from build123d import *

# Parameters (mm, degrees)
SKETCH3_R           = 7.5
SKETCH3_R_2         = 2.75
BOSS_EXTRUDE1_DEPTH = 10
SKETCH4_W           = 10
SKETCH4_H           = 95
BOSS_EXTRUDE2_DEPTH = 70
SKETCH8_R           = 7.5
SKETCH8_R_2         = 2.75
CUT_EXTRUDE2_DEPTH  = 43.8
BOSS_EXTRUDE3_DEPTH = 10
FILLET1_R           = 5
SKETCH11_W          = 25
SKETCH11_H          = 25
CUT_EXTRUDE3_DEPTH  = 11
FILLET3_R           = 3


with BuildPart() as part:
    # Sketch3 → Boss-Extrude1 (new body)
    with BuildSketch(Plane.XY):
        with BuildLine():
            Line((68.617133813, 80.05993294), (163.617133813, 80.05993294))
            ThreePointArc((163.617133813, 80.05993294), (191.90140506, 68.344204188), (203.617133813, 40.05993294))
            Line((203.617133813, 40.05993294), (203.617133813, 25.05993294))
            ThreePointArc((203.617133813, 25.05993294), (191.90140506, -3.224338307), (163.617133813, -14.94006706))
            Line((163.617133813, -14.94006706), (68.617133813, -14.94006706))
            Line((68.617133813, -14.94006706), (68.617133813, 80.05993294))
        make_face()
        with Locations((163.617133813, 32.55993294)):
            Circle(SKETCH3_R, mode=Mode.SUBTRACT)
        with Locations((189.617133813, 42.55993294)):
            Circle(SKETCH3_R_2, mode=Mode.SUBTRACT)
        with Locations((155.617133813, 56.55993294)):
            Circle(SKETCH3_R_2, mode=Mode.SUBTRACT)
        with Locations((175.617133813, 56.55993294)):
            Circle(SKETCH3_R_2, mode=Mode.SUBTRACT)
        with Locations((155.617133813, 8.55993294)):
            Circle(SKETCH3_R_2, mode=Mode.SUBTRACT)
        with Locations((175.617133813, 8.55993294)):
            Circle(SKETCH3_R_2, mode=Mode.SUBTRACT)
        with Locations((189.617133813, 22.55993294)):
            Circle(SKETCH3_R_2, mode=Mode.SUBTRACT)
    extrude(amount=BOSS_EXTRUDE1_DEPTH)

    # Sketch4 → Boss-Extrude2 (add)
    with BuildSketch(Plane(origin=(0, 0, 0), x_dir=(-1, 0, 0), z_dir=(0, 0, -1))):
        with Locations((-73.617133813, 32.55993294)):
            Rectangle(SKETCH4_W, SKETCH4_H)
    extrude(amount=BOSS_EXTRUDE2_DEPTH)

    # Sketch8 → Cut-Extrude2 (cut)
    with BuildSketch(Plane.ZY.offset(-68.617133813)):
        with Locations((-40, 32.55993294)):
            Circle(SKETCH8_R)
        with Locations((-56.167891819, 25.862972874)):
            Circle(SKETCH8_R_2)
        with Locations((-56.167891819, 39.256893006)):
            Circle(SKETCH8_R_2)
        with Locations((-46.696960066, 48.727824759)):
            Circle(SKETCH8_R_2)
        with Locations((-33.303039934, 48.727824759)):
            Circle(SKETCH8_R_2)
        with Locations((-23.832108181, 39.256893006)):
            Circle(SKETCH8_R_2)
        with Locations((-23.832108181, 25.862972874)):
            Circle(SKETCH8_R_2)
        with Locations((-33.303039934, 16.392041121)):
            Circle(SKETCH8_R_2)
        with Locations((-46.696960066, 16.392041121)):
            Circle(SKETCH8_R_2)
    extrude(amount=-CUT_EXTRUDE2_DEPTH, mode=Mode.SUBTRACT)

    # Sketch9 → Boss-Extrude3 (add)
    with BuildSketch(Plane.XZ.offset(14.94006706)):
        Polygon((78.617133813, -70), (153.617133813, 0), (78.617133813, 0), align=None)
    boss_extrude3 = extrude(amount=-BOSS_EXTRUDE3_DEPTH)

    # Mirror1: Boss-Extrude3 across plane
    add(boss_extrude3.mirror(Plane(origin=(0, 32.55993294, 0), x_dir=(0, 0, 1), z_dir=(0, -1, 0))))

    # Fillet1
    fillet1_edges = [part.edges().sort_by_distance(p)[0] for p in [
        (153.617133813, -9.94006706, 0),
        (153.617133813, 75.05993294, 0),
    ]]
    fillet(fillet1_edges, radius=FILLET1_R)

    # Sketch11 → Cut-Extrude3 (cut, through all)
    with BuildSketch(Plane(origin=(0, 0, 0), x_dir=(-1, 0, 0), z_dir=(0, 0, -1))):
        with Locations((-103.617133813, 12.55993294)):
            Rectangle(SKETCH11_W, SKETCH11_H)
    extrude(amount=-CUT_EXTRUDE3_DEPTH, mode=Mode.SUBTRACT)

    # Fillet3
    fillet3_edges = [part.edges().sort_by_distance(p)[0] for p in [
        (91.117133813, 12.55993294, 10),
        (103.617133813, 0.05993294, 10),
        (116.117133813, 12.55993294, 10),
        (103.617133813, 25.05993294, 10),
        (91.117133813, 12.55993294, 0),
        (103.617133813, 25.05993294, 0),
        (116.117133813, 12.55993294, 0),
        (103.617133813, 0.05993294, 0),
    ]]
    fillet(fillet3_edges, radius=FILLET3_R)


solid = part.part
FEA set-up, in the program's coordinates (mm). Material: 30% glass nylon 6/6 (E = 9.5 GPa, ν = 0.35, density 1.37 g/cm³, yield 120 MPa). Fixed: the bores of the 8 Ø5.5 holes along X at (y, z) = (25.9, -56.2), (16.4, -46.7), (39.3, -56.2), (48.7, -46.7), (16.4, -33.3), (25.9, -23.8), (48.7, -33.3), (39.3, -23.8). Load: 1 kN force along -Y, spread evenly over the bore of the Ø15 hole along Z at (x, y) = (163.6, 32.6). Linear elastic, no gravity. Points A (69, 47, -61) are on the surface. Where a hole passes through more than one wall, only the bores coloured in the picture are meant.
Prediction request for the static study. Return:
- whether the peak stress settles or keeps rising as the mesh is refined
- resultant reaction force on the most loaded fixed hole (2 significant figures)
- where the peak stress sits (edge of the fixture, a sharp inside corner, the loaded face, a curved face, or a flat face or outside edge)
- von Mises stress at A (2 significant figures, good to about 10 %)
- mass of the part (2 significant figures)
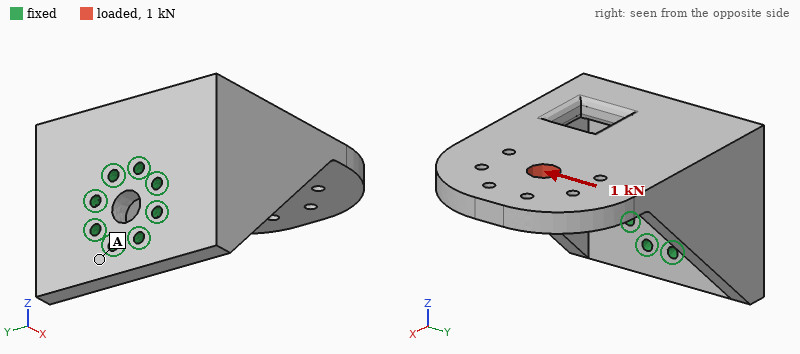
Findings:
keeps rising
1.1 kN
edge of the fixture
6.4 MPa
310 g
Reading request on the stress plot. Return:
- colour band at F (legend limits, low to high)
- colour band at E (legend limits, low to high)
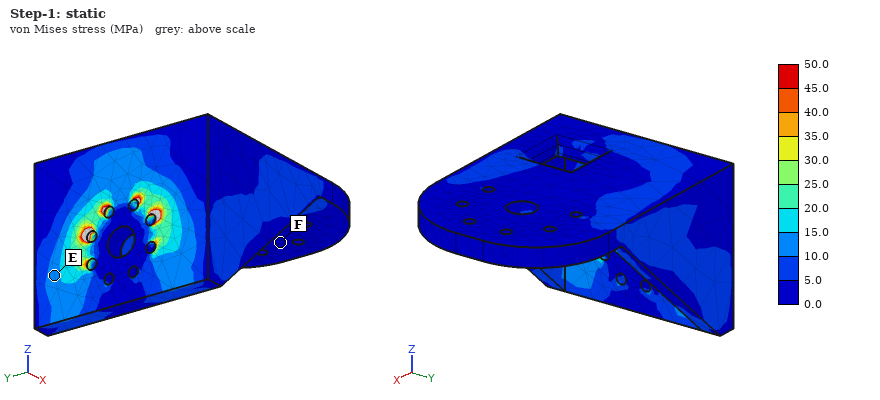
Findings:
0.0 to 5.0 MPa
10.0 to 15.0 MPa
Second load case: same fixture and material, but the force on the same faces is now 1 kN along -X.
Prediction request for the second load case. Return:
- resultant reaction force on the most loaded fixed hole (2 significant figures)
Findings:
520 N
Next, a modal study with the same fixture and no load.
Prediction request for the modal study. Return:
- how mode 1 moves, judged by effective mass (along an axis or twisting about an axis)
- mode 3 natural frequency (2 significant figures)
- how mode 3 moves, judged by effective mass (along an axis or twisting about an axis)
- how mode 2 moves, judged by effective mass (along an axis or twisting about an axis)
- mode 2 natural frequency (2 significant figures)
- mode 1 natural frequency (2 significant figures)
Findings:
along Y
1300 Hz
along X
along Z
500 Hz
480 Hz
